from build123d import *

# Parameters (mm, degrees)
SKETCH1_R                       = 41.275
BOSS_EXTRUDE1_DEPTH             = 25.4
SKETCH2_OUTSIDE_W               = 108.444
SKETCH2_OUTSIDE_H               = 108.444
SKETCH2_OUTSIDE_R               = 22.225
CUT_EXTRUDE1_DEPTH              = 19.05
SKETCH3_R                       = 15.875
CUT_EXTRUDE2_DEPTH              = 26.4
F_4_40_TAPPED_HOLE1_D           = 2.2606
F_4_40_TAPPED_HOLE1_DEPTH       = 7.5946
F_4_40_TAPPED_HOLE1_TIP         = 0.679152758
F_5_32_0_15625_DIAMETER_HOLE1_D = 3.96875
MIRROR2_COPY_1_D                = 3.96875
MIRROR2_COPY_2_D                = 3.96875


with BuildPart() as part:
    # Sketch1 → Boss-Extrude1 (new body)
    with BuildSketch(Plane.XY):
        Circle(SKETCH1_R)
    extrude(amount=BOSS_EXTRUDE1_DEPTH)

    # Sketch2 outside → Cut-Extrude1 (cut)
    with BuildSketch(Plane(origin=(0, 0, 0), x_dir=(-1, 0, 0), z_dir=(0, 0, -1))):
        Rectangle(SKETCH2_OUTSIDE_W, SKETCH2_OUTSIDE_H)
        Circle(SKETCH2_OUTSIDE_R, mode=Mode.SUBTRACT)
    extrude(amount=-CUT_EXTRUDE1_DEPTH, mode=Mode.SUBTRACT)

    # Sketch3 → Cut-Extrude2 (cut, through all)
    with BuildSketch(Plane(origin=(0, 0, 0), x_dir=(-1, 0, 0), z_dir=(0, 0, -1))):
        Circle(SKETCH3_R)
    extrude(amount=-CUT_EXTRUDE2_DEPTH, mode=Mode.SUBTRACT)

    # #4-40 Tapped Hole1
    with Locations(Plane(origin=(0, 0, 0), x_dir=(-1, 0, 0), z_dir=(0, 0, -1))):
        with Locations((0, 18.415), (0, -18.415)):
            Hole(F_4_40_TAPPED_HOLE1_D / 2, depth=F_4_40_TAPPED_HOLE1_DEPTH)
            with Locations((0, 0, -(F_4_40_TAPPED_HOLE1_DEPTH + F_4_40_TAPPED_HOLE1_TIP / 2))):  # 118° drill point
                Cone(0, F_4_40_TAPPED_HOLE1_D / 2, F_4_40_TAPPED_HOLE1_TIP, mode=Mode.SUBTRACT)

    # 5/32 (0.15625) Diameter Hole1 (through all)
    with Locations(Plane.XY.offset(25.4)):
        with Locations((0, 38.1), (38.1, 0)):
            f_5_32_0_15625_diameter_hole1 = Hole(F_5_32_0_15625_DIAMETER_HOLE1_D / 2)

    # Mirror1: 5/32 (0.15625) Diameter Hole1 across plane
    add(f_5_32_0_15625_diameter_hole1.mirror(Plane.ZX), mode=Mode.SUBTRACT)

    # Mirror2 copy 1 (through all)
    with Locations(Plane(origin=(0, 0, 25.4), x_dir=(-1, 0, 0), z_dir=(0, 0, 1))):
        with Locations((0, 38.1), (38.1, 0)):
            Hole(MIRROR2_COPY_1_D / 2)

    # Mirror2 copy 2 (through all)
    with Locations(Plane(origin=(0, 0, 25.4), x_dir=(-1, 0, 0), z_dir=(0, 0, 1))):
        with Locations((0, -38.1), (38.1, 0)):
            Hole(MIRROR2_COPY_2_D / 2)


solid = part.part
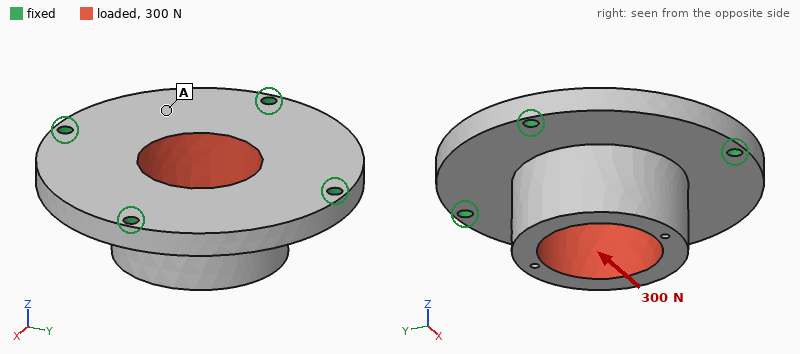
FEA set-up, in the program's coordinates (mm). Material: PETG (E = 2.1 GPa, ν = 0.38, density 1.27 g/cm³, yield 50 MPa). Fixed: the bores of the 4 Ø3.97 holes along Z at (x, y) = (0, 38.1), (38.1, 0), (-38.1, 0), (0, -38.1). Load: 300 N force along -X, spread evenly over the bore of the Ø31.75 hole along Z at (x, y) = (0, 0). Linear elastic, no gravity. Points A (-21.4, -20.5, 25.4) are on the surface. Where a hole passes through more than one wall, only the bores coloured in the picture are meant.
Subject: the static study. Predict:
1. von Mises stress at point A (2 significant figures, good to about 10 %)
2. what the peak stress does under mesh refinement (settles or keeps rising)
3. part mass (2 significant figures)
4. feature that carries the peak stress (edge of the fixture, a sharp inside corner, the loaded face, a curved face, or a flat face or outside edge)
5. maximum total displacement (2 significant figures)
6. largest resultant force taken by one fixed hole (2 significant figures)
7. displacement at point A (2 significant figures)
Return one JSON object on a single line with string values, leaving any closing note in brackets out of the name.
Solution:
{"von Mises stress at point A": "0.53 MPa", "what the peak stress does under mesh refinement": "keeps rising", "part mass": "55 g", "feature that carries the peak stress": "edge of the fixture", "maximum total displacement": "45 µm", "largest resultant force taken by one fixed hole": "99 N", "displacement at point A": "18 µm"}
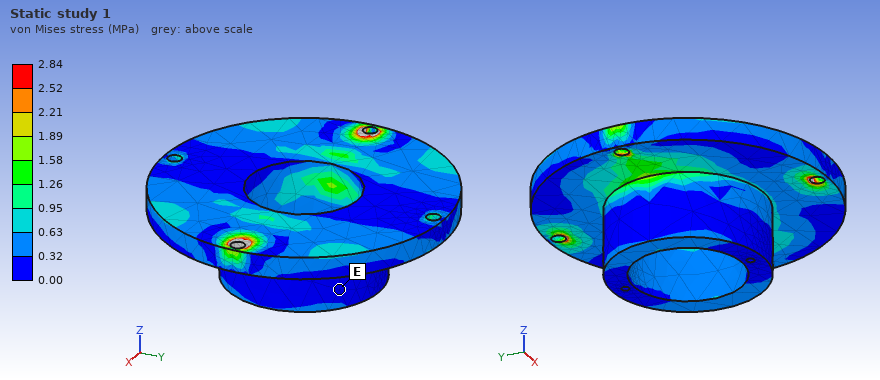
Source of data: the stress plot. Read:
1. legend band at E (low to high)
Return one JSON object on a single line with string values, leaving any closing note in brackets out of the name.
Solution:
{"legend band at E": "0.00 to 0.32 MPa"}
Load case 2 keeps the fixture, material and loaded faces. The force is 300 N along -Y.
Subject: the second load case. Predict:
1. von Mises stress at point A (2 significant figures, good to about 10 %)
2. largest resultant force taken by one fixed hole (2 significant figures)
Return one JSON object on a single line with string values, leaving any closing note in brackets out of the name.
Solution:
{"von Mises stress at point A": "0.52 MPa", "largest resultant force taken by one fixed hole": "99 N"}
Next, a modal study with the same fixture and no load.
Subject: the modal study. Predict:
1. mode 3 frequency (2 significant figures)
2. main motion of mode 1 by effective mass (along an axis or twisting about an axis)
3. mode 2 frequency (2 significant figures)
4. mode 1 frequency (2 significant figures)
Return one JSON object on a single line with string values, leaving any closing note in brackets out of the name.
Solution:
{"mode 3 frequency": "2100 Hz", "main motion of mode 1 by effective mass": "along Z", "mode 2 frequency": "2100 Hz", "mode 1 frequency": "1800 Hz"}
